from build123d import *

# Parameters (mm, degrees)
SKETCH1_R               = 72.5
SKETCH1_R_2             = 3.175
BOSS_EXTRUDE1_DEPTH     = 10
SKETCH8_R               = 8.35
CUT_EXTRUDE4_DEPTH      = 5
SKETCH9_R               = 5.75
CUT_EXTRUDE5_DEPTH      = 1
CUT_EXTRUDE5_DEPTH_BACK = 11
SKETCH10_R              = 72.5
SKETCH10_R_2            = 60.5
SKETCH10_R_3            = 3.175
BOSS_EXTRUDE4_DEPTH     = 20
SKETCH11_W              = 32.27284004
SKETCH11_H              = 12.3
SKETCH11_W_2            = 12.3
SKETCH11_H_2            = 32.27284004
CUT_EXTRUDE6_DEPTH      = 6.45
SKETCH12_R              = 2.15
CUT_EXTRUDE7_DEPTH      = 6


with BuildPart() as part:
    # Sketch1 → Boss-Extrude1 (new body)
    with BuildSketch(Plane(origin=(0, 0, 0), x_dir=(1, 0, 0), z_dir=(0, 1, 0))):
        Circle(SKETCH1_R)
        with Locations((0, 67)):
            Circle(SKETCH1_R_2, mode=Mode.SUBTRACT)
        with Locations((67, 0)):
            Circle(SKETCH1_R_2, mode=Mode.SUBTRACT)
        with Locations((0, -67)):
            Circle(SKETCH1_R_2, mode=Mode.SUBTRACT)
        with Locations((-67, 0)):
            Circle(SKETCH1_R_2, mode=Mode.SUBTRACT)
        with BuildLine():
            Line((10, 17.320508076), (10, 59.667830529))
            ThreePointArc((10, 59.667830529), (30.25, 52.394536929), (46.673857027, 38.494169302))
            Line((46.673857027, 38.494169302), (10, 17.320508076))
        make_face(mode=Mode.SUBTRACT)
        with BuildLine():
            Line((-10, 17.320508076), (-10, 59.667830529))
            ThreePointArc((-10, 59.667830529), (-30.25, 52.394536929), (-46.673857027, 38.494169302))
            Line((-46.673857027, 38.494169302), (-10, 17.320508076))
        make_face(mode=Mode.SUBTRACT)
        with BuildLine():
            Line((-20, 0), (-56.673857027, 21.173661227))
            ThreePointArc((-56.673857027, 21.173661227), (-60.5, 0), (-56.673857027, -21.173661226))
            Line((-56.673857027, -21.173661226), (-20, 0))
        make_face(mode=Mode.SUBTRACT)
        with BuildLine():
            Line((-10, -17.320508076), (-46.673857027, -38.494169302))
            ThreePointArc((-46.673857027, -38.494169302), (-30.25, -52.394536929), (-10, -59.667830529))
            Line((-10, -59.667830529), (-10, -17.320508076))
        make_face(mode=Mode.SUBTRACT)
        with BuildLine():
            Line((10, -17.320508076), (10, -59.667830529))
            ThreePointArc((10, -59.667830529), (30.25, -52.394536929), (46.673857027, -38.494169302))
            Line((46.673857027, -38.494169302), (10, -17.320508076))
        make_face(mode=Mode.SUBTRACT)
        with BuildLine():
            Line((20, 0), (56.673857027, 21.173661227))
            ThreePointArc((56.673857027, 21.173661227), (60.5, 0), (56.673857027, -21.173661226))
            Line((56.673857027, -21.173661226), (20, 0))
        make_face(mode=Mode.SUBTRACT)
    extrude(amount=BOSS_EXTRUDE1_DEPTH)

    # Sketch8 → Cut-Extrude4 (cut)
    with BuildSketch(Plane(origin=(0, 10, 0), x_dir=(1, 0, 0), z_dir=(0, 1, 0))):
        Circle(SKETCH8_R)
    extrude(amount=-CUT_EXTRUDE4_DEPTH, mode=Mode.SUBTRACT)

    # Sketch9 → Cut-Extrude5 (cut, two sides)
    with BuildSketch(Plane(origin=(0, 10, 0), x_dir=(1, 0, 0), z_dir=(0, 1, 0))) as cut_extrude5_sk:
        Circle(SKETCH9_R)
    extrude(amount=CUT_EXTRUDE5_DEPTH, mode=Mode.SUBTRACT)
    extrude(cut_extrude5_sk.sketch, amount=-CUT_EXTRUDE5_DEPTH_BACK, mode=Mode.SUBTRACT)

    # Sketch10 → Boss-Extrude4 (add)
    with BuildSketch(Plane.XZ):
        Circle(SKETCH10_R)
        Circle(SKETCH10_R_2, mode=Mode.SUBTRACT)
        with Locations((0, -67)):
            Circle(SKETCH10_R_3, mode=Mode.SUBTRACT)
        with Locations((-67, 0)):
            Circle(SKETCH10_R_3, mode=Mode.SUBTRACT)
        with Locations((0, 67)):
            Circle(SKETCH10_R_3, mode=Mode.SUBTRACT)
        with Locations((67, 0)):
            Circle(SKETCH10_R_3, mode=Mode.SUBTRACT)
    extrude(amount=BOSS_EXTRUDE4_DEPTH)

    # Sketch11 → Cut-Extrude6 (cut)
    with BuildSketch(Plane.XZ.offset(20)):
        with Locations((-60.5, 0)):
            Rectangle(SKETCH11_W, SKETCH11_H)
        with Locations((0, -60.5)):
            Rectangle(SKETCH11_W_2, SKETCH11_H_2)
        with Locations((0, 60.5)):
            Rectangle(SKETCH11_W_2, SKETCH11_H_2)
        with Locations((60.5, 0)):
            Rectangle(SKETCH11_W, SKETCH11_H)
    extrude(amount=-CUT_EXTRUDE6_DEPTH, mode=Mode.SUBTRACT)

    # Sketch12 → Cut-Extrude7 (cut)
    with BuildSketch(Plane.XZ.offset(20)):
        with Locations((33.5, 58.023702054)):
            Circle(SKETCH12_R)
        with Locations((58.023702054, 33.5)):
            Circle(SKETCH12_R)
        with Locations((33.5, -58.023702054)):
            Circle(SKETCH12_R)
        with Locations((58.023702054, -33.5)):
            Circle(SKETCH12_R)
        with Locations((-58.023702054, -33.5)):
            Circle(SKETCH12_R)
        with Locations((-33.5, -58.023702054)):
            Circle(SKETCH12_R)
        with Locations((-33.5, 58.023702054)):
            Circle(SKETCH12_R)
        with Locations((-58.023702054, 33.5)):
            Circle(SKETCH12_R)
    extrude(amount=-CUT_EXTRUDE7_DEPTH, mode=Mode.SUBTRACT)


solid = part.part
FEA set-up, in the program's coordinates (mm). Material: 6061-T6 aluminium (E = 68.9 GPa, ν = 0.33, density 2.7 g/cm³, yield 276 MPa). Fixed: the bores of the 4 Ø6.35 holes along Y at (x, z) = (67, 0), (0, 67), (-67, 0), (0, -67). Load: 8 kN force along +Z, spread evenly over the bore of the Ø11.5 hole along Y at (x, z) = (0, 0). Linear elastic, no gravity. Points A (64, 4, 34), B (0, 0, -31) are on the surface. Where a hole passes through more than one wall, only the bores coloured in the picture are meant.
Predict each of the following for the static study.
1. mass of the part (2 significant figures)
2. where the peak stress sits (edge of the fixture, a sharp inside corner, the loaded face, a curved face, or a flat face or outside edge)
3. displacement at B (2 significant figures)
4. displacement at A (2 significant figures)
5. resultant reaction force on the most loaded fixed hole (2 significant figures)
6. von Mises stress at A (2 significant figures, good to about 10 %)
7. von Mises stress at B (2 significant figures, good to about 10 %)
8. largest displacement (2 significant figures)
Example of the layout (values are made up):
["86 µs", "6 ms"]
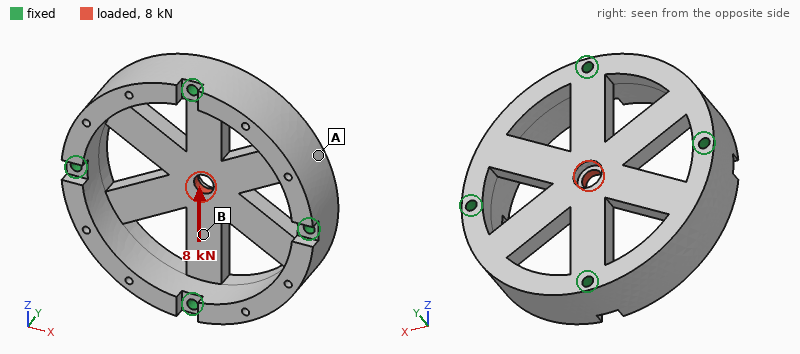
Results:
["550 g", "a sharp inside corner", "10 µm", "4.5 µm", "2.8 kN", "5.4 MPa", "22 MPa", "20 µm"]
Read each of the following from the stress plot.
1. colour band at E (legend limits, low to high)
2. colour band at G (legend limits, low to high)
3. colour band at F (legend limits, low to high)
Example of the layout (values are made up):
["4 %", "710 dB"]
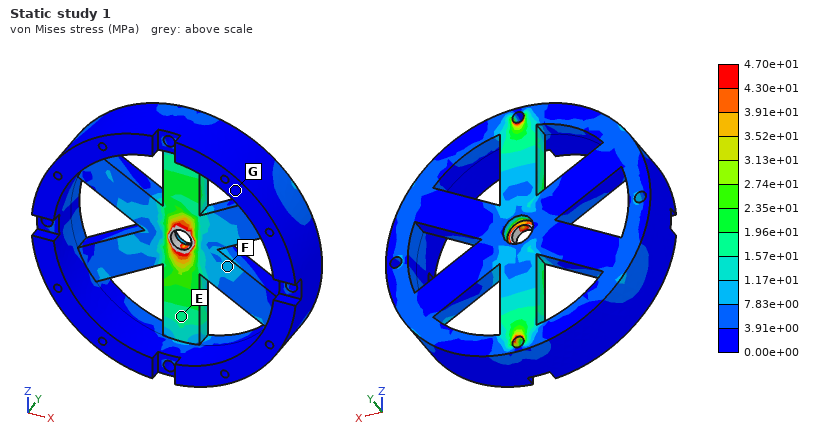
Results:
["1.57e+01 to 1.96e+01 MPa", "0.00e+00 to 3.91e+00 MPa", "7.83e+00 to 1.17e+01 MPa"]
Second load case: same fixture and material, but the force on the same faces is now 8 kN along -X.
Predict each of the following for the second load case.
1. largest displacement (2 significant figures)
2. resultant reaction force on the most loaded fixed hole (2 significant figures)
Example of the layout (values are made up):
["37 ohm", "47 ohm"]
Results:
["32 µm", "2.8 kN"]
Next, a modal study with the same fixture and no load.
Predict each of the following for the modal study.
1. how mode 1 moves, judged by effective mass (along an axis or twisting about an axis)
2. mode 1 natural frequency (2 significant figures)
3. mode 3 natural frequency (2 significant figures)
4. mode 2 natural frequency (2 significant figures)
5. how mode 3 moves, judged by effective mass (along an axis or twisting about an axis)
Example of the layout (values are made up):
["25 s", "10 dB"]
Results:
["along Y", "3700 Hz", "7400 Hz", "7100 Hz", "twisting about X"]
